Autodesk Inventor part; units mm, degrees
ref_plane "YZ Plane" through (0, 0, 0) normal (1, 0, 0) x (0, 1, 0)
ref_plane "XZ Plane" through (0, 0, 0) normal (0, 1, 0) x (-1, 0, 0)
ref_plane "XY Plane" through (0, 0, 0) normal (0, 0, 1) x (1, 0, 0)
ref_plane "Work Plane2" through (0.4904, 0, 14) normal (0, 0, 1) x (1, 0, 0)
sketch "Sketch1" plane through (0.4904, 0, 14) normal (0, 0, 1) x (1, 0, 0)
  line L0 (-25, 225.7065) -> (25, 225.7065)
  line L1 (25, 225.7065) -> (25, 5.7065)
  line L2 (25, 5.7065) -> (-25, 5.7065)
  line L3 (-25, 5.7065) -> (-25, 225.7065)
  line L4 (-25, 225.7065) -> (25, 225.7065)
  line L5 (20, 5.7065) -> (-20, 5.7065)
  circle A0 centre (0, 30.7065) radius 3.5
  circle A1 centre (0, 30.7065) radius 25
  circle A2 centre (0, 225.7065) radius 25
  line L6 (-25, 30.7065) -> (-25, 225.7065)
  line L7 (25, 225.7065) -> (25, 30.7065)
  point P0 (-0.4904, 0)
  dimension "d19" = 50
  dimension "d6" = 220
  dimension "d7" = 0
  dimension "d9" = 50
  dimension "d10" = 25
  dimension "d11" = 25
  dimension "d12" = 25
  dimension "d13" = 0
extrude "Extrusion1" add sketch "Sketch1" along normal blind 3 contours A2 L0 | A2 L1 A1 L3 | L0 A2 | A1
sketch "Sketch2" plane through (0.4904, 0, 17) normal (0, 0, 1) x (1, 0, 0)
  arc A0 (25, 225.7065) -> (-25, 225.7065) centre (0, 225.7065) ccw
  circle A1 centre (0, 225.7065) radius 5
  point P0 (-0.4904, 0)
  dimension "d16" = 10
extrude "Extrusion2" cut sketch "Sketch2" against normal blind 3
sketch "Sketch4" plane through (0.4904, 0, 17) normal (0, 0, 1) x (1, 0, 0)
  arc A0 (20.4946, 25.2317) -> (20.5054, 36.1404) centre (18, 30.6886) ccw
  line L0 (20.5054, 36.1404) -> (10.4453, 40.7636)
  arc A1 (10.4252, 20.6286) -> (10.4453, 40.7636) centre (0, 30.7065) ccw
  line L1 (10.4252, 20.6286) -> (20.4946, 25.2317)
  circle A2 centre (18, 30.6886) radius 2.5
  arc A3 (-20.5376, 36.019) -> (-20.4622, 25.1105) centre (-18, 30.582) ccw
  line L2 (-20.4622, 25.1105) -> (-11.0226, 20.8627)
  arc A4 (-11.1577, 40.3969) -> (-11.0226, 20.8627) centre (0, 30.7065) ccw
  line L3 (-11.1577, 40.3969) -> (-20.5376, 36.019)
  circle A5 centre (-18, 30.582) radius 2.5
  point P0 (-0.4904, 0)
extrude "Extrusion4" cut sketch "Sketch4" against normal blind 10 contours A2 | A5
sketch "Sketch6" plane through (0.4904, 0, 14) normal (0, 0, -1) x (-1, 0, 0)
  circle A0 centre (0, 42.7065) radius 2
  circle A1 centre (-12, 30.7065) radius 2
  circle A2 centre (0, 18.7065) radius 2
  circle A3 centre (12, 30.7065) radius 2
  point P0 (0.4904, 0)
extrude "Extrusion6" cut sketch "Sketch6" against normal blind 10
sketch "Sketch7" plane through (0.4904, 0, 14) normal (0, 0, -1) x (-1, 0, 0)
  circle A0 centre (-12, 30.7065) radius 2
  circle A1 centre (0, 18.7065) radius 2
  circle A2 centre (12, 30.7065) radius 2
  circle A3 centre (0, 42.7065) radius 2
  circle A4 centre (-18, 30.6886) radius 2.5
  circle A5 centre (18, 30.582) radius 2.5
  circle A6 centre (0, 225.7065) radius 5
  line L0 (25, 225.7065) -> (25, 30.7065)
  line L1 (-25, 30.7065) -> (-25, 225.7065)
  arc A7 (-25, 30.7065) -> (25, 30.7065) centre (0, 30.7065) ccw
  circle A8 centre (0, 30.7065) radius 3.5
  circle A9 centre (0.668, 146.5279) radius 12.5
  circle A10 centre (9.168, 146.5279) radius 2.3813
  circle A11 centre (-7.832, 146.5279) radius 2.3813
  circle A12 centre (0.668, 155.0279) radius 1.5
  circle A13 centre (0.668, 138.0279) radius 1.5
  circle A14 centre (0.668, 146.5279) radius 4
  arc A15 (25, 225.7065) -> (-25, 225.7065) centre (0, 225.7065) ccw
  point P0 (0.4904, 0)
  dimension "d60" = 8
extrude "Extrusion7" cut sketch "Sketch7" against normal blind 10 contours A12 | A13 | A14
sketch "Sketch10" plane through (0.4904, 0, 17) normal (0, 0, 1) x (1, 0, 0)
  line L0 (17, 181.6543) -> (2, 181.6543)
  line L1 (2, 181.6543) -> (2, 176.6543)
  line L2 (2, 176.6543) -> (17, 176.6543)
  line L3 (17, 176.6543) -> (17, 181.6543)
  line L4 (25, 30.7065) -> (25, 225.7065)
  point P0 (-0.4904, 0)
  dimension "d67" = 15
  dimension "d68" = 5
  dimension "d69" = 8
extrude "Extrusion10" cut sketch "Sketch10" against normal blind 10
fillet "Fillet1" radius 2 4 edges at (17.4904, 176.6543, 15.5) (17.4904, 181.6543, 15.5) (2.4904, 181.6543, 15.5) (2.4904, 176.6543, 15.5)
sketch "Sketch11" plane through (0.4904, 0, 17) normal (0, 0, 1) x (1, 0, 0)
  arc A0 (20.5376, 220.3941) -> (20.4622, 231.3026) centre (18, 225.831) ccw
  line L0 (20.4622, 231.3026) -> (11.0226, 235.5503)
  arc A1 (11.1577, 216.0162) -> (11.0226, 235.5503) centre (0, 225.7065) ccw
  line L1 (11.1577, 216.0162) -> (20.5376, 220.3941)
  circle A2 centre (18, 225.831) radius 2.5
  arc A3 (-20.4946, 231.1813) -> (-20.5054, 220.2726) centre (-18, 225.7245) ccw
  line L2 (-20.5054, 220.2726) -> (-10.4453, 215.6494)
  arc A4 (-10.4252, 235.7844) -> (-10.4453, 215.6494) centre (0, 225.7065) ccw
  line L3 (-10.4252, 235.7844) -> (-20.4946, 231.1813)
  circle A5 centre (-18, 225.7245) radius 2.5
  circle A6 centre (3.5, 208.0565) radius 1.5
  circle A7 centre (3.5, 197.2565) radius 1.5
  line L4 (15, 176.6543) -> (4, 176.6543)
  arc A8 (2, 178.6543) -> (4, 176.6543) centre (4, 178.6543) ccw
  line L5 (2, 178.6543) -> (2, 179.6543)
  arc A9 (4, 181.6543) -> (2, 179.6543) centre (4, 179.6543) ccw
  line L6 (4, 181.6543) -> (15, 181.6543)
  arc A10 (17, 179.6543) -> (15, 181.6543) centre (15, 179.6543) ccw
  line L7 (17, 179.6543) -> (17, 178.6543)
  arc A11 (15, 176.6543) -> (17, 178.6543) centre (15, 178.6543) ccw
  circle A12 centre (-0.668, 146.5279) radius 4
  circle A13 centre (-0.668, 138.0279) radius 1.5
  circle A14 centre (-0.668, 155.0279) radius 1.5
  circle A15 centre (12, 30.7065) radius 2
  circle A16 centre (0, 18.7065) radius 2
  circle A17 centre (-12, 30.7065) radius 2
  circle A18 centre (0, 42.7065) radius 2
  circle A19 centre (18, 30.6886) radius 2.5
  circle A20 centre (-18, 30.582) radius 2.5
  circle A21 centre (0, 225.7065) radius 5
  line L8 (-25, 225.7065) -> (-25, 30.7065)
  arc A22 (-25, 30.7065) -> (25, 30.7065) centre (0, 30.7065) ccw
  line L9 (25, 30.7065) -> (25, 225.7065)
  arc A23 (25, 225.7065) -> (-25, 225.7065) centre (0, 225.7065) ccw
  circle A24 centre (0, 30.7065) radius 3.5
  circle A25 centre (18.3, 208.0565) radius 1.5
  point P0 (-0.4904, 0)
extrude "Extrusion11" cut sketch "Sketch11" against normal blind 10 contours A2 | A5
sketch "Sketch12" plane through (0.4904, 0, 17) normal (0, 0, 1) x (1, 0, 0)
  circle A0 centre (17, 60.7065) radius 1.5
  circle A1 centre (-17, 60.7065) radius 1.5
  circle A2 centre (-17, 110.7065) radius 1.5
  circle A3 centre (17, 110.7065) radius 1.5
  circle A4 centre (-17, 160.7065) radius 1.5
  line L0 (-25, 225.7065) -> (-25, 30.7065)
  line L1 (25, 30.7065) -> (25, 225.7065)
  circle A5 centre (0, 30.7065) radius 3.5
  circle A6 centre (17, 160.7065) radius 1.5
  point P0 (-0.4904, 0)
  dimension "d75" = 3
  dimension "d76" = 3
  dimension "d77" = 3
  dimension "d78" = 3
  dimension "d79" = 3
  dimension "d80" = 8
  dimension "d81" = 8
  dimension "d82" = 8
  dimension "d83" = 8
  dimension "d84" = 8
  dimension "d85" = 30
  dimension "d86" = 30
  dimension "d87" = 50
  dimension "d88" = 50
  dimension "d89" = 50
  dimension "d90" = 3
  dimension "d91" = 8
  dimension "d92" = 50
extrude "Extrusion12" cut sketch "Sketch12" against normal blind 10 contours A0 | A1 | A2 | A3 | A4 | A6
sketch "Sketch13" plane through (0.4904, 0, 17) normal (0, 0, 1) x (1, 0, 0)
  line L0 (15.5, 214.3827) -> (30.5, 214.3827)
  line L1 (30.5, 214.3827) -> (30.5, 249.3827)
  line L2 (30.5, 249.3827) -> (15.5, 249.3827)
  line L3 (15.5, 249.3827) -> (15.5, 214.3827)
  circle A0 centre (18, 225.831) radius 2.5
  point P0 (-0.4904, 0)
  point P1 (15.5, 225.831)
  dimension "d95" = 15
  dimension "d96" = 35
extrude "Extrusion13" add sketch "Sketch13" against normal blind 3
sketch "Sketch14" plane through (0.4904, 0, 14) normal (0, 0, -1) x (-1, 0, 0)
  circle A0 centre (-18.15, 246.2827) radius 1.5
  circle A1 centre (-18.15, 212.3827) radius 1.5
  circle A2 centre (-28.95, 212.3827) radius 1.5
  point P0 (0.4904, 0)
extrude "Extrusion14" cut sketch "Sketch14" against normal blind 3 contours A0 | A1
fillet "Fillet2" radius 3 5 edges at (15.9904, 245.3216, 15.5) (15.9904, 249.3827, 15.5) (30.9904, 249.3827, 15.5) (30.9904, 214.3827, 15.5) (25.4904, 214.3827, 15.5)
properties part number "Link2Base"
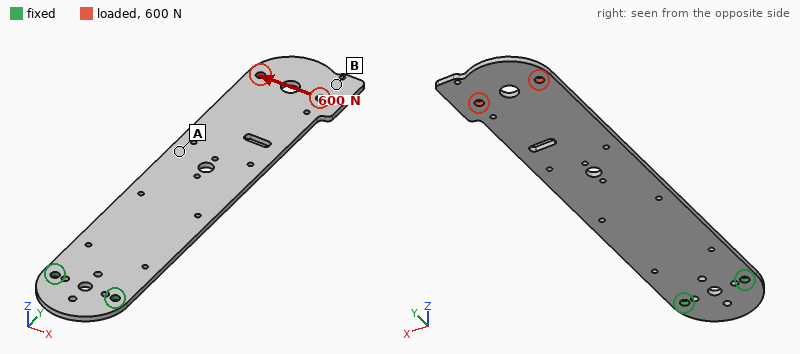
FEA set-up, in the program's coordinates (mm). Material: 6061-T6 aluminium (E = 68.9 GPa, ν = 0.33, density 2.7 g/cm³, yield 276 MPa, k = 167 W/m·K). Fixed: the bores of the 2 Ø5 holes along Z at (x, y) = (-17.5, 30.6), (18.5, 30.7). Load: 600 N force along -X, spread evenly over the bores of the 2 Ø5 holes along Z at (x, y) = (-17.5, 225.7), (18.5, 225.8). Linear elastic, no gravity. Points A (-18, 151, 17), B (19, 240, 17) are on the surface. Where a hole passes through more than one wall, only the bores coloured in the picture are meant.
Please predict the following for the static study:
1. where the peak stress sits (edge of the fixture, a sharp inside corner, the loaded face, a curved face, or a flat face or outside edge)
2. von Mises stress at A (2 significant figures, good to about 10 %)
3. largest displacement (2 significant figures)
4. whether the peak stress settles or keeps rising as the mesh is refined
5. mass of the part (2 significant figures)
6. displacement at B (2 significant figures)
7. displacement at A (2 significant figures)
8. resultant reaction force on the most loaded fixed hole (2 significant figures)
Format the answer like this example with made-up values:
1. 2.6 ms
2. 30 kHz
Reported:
1. edge of the fixture
2. 27 MPa
3. 0.91 mm
4. keeps rising
5. 94 g
6. 0.85 mm
7. 0.36 mm
8. 3.1 kN
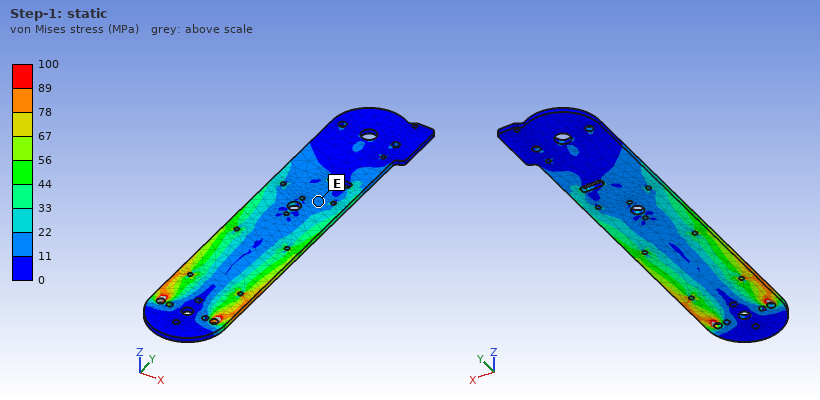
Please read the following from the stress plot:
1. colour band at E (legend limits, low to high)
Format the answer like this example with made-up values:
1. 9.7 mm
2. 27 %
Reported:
1. 11 to 22 MPa
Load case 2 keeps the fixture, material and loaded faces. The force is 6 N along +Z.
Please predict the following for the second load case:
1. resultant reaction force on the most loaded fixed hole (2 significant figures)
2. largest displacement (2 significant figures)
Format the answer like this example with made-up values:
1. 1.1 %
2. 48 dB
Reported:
1. 3.1 N
2. 2.4 mm
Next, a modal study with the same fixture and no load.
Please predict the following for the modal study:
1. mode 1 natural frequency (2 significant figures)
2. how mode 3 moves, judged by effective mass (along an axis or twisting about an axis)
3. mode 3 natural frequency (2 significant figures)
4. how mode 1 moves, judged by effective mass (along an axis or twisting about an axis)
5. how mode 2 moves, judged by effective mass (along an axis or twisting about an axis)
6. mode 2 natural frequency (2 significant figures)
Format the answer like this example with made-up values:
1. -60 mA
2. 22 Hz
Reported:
1. 51 Hz
2. twisting about Y
3. 430 Hz
4. along Z
5. along Z
6. 310 Hz
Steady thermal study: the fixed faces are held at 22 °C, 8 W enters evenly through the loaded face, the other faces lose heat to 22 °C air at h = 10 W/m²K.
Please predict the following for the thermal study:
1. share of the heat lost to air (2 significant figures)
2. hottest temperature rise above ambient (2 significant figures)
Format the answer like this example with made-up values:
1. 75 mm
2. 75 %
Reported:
1. 57 %
2. 40 K
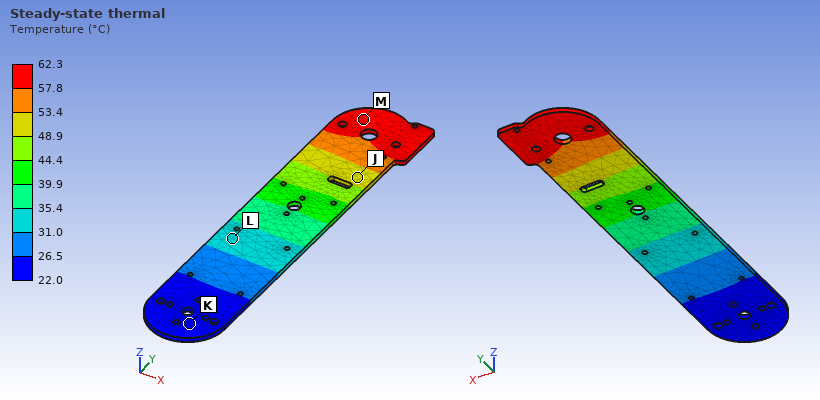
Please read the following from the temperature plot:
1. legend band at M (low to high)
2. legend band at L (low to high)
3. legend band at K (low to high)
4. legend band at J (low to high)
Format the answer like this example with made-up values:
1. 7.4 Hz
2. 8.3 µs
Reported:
1. 57.8 to 62.3 °C
2. 31.0 to 35.4 °C
3. 22.0 to 26.5 °C
4. 48.9 to 53.4 °C
